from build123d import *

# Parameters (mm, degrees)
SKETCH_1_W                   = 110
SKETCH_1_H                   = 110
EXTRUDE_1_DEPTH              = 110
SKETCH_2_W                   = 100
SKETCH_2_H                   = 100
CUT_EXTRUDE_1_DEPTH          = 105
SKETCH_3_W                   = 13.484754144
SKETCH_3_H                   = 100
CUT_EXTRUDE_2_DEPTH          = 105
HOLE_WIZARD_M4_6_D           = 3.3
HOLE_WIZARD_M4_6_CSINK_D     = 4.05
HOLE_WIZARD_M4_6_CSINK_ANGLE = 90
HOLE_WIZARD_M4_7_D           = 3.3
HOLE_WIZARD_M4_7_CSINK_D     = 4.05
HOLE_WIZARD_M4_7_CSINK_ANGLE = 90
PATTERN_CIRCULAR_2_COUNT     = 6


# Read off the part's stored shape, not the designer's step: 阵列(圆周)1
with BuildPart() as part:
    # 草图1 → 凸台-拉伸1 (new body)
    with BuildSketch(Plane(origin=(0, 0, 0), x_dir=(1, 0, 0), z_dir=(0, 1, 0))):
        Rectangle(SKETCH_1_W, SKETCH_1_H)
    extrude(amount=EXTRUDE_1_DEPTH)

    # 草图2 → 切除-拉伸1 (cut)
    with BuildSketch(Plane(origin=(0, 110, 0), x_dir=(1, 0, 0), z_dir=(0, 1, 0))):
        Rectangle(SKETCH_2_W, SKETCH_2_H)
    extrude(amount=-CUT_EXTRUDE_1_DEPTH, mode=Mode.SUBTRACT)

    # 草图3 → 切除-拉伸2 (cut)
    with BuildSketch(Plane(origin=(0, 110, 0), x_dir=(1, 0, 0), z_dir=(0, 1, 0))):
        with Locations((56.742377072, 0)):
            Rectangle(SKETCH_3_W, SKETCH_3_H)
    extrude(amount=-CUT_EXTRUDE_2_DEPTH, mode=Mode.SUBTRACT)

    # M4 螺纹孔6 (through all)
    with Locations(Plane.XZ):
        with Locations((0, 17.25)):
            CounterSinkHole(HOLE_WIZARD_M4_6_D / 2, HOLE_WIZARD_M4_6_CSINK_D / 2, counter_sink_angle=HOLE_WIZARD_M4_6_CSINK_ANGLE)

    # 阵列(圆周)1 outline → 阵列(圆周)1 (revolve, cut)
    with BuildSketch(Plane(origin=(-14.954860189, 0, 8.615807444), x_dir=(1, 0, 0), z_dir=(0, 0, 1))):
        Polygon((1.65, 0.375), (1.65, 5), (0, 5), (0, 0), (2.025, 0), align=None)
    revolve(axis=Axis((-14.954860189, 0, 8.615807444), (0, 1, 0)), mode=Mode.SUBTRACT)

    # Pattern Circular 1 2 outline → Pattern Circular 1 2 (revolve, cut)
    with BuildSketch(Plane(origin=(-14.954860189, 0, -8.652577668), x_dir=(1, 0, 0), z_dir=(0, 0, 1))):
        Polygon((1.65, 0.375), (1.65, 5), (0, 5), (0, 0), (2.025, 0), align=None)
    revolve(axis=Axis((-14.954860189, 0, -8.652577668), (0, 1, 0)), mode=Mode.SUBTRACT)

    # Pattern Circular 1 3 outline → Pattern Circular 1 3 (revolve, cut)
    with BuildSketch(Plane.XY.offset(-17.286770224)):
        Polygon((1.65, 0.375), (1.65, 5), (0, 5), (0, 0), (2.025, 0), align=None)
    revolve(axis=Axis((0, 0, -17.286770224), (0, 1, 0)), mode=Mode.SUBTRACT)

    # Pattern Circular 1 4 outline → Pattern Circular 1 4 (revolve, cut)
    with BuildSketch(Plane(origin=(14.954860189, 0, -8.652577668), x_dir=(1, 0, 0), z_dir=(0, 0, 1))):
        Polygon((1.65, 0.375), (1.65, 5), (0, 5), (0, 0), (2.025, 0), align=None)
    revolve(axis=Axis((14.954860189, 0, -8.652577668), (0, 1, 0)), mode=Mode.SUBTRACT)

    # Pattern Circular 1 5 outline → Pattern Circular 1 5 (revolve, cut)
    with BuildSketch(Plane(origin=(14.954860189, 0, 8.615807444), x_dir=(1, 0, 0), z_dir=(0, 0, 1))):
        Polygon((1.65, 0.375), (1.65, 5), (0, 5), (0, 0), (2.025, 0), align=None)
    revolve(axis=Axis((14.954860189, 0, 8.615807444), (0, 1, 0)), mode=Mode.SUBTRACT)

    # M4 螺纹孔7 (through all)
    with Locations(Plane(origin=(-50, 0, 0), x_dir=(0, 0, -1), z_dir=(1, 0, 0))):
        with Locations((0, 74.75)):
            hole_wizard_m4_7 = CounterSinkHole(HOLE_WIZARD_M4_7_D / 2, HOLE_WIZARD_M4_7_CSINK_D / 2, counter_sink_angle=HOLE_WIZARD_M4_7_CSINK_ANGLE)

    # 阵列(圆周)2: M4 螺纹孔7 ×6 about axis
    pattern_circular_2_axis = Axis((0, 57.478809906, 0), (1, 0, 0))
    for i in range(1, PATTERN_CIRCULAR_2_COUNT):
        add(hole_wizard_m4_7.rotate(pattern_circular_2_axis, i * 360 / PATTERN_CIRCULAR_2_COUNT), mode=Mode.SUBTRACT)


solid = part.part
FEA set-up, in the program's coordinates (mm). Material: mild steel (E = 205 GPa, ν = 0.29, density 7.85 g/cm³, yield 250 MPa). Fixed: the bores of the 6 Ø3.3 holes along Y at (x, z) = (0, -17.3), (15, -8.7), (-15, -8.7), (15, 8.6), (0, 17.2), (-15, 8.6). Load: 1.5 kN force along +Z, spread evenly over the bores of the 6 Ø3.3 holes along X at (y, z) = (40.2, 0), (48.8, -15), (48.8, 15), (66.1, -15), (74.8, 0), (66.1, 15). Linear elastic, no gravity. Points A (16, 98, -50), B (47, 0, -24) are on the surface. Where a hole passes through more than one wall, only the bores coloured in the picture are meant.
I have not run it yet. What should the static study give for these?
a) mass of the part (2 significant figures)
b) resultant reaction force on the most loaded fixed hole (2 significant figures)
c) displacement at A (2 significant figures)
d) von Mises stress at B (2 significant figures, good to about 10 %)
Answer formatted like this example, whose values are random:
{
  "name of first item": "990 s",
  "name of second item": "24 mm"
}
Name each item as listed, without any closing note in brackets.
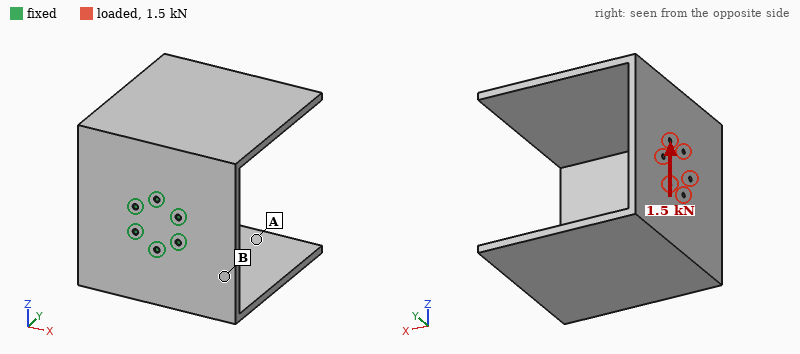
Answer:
{
  "mass of the part": "1.8 kg",
  "resultant reaction force on the most loaded fixed hole": "1.4 kN",
  "displacement at A": "0.35 mm",
  "von Mises stress at B": "31 MPa"
}
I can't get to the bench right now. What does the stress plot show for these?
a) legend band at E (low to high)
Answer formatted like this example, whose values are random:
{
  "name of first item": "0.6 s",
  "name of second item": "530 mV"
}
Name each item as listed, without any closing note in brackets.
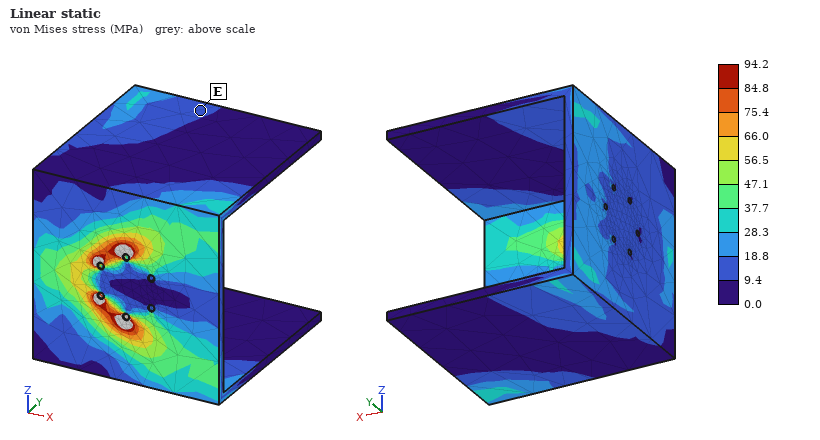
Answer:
{
  "legend band at E": "9.4 to 18.8 MPa"
}
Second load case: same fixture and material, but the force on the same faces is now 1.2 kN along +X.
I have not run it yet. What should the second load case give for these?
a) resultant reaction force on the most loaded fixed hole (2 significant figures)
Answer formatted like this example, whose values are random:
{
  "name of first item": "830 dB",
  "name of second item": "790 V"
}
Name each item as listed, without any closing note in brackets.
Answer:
{
  "resultant reaction force on the most loaded fixed hole": "850 N"
}
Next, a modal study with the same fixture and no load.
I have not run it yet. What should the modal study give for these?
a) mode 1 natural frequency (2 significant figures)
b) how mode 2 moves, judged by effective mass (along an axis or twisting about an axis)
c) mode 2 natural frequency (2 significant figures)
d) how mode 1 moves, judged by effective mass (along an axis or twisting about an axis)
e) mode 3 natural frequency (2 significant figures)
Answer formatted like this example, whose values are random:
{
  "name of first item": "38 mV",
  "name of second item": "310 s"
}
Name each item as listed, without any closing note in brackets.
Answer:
{
  "mode 1 natural frequency": "280 Hz",
  "how mode 2 moves, judged by effective mass": "along X",
  "mode 2 natural frequency": "340 Hz",
  "how mode 1 moves, judged by effective mass": "along Z",
  "mode 3 natural frequency": "570 Hz"
}
